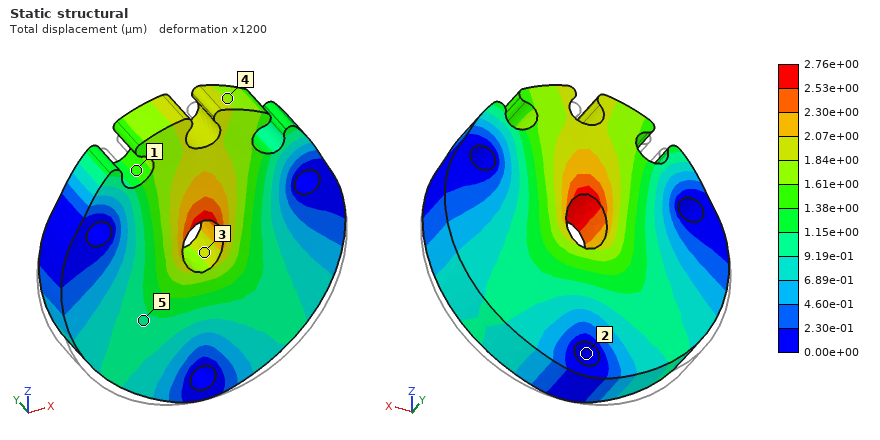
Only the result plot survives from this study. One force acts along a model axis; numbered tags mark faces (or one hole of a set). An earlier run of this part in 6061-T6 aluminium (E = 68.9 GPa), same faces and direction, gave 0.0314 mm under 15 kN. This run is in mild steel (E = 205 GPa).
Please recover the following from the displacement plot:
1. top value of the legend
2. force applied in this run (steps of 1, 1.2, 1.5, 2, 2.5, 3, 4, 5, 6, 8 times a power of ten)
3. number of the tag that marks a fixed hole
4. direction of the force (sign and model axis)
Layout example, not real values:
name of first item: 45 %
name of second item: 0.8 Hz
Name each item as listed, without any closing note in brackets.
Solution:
top value of the legend: 2.76e+00 µm
force applied in this run: 4 kN
number of the tag that marks a fixed hole: 2
direction of the force: +Z
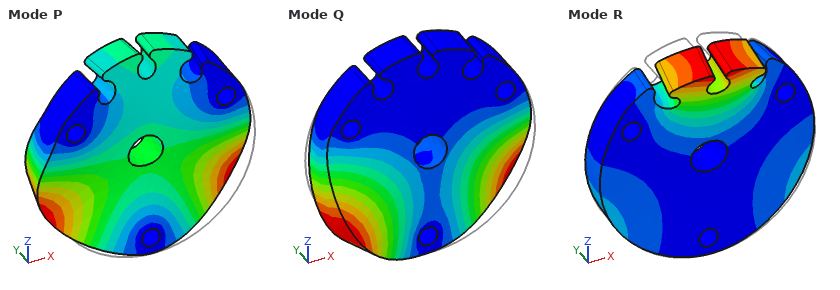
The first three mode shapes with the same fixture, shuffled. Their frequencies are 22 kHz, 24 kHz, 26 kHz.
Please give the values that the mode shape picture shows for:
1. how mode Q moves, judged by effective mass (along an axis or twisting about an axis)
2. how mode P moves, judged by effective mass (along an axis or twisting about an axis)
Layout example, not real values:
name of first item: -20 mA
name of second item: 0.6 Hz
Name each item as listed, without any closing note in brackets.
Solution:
how mode Q moves, judged by effective mass: twisting about Z
how mode P moves, judged by effective mass: along Y
